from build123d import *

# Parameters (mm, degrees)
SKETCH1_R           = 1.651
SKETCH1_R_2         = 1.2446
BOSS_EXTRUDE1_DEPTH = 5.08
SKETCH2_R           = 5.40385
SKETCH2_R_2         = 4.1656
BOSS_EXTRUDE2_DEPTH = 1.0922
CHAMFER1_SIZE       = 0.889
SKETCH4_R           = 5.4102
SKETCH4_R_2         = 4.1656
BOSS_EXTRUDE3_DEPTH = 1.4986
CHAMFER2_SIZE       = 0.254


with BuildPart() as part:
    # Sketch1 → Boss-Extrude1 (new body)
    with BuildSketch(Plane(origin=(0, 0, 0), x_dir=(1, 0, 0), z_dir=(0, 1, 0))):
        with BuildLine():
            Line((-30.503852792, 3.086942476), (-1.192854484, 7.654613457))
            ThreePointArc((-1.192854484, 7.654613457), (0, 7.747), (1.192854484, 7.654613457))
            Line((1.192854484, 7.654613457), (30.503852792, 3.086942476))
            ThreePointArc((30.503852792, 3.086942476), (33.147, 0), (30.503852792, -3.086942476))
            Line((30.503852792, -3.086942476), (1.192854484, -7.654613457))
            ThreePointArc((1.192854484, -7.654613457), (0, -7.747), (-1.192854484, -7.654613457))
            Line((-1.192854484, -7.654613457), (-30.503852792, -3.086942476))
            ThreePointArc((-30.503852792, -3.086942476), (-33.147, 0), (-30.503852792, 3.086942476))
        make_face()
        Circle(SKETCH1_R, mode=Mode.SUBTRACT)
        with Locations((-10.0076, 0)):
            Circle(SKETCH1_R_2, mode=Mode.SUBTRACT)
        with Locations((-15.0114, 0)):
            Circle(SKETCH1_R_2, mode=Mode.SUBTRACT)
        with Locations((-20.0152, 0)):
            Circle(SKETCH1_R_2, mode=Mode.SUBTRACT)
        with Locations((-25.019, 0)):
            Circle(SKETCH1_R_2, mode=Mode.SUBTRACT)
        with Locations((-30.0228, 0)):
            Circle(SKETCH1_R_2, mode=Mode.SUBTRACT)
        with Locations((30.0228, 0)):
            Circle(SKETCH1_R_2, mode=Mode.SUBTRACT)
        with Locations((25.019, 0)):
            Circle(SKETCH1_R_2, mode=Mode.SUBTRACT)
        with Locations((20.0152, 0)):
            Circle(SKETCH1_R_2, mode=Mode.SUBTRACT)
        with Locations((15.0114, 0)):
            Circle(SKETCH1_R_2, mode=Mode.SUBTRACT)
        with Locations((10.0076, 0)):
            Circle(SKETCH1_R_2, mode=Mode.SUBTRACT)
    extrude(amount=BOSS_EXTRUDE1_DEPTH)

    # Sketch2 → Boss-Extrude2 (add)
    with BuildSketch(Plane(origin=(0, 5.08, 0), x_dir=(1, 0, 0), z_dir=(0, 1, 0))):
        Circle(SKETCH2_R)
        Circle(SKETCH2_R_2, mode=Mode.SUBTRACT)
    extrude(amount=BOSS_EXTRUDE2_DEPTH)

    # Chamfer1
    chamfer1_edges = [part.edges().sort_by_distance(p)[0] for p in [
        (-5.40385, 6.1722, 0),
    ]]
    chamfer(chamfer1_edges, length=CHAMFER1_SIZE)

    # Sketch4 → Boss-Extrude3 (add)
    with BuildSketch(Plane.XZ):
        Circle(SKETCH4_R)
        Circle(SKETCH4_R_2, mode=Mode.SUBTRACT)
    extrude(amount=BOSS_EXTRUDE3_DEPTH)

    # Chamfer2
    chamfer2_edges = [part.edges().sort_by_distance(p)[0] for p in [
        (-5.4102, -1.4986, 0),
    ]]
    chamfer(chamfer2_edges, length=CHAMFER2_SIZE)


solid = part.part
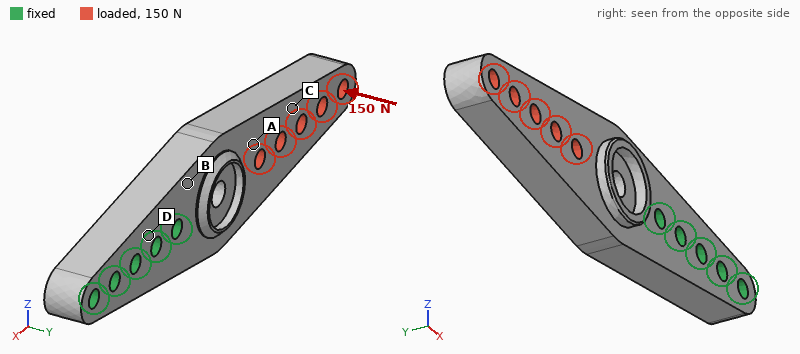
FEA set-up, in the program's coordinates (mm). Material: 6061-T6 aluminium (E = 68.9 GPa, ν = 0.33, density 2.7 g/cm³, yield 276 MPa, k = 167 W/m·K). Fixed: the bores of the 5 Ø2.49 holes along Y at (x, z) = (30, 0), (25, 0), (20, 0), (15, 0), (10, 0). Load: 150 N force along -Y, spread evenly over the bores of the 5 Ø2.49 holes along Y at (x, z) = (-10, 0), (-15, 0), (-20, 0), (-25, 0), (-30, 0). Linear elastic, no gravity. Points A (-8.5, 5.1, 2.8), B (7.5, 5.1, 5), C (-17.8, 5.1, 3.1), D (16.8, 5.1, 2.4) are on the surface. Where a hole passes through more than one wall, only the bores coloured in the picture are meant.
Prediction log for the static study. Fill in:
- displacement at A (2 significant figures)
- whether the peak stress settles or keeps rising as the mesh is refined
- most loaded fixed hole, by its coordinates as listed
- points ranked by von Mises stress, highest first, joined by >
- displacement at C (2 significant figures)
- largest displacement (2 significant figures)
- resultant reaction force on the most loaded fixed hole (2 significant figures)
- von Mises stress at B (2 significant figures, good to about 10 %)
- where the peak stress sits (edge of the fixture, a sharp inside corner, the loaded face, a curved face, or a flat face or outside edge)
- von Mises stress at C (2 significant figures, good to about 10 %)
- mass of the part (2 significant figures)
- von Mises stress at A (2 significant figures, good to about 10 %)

0.066 mm
keeps rising
(10, 0)
B > A > C > D
0.13 mm
0.24 mm
380 N
57 MPa
edge of the fixture
20 MPa
8.9 g
37 MPa
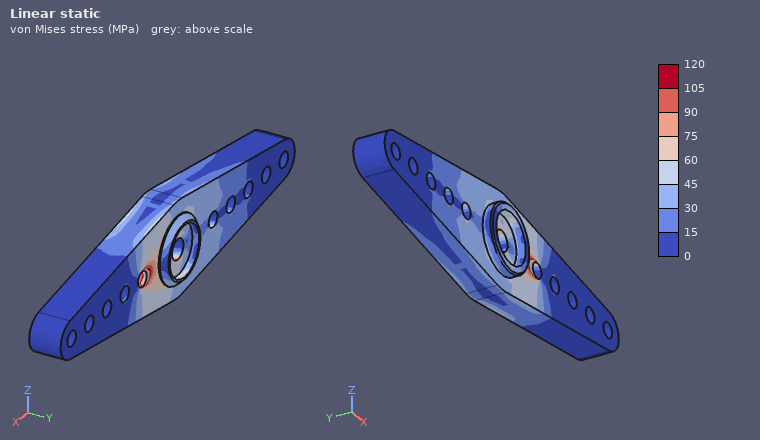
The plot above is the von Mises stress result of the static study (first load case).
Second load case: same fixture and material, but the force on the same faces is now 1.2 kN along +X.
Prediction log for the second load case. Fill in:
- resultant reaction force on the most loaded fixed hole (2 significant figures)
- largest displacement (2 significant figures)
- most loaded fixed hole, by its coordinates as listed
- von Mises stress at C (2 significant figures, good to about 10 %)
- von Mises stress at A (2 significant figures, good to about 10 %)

850 N
11 µm
(10, 0)
19 MPa
21 MPa
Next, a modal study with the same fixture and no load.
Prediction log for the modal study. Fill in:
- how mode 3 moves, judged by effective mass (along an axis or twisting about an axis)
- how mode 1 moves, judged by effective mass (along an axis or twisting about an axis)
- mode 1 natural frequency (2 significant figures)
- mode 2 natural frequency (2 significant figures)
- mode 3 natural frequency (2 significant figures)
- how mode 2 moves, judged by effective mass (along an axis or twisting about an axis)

along Y
along Y
3000 Hz
6000 Hz
14 kHz
along Z
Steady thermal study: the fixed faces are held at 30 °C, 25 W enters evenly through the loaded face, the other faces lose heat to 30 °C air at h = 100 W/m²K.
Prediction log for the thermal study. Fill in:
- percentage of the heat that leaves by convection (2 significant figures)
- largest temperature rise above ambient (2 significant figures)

21 %
69 K
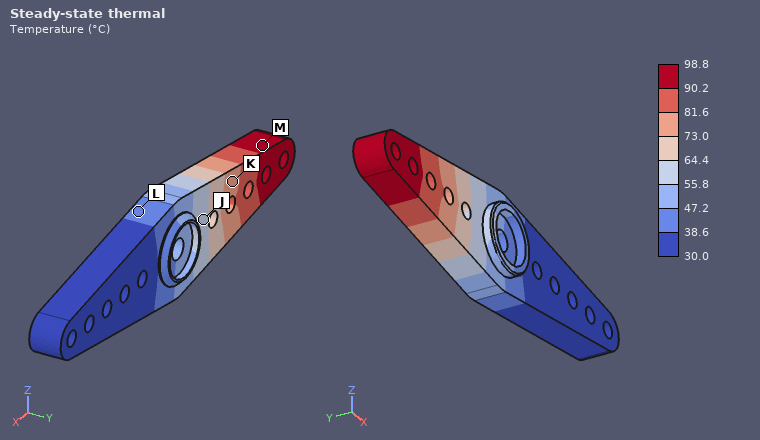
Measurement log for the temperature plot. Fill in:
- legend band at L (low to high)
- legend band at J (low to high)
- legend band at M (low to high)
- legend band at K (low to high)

38.6 to 47.2 °C
55.8 to 64.4 °C
90.2 to 98.8 °C
73.0 to 81.6 °C
